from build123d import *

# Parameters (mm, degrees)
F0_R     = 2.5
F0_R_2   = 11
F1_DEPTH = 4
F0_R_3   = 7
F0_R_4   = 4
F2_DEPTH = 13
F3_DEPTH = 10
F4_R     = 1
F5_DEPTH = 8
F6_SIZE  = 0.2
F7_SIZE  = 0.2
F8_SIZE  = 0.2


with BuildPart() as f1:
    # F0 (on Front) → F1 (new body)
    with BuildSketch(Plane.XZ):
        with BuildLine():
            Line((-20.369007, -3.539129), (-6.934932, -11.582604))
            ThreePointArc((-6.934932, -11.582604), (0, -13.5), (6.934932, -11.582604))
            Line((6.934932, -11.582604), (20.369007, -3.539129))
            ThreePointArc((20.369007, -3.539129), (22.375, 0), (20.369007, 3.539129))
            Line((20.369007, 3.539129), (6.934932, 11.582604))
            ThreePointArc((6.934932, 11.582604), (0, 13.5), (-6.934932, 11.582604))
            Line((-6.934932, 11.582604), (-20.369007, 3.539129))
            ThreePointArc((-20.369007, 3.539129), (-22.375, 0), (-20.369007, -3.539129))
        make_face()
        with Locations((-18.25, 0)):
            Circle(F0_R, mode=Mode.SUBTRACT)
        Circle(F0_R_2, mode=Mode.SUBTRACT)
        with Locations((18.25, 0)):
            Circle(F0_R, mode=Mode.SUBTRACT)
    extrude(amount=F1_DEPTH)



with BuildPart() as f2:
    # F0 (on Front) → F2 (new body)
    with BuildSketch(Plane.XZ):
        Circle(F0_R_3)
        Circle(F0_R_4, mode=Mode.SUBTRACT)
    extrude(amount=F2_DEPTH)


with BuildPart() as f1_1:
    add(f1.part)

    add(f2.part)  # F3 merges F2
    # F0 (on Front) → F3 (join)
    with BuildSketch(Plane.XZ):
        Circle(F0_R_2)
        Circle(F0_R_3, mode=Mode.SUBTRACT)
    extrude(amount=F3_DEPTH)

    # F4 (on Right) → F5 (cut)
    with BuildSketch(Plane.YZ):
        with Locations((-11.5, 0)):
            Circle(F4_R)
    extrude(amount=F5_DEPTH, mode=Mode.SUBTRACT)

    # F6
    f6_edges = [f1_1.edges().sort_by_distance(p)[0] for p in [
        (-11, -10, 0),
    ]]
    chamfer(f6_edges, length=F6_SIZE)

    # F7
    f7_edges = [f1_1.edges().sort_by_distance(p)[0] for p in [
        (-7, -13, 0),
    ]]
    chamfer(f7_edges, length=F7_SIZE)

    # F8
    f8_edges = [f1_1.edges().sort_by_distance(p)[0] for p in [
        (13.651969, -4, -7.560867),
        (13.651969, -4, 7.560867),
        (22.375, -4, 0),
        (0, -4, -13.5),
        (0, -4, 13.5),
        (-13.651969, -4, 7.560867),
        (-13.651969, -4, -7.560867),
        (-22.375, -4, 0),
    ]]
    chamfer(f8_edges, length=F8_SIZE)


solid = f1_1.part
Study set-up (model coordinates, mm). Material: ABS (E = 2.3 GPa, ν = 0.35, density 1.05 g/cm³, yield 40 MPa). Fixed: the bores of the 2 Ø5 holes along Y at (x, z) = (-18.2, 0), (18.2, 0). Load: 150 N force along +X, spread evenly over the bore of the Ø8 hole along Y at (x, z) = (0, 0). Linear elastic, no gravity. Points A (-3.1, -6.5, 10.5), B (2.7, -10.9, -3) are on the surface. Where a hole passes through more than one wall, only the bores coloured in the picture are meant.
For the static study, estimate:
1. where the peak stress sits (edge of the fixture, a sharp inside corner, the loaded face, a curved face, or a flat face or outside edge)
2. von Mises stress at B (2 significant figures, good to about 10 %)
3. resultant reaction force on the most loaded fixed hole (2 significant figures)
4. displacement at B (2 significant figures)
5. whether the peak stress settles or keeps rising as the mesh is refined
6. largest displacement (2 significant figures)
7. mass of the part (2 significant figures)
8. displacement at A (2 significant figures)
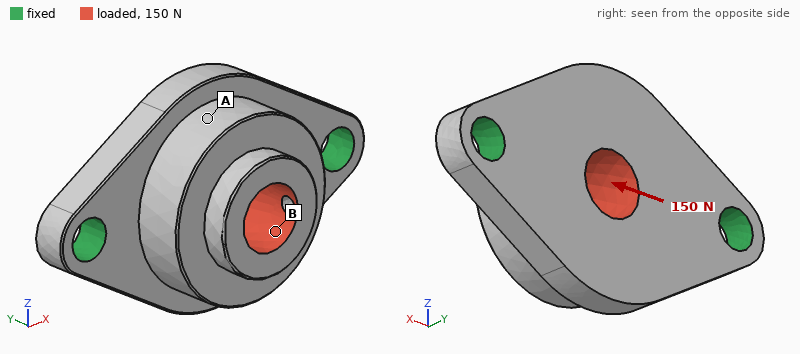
edge of the fixture
0.93 MPa
79 N
16 µm
keeps rising
19 µm
5.3 g
9.8 µm
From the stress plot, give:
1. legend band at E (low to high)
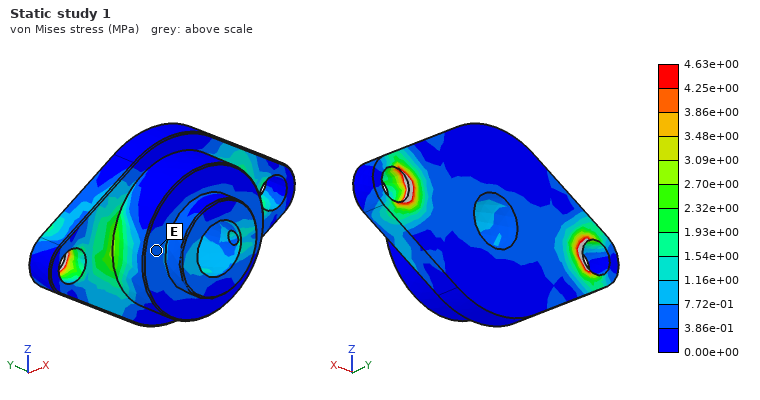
3.86e-01 to 7.72e-01 MPa
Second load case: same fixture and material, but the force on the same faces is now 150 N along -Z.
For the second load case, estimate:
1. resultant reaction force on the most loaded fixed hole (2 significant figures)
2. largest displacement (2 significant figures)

75 N
0.14 mm
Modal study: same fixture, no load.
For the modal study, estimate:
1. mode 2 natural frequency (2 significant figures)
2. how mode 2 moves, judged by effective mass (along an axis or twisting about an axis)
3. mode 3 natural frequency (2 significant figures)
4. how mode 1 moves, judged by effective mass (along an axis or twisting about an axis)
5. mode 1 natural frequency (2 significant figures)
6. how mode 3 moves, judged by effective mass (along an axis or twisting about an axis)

4300 Hz
along Y
7400 Hz
along Z
2600 Hz
along Z
